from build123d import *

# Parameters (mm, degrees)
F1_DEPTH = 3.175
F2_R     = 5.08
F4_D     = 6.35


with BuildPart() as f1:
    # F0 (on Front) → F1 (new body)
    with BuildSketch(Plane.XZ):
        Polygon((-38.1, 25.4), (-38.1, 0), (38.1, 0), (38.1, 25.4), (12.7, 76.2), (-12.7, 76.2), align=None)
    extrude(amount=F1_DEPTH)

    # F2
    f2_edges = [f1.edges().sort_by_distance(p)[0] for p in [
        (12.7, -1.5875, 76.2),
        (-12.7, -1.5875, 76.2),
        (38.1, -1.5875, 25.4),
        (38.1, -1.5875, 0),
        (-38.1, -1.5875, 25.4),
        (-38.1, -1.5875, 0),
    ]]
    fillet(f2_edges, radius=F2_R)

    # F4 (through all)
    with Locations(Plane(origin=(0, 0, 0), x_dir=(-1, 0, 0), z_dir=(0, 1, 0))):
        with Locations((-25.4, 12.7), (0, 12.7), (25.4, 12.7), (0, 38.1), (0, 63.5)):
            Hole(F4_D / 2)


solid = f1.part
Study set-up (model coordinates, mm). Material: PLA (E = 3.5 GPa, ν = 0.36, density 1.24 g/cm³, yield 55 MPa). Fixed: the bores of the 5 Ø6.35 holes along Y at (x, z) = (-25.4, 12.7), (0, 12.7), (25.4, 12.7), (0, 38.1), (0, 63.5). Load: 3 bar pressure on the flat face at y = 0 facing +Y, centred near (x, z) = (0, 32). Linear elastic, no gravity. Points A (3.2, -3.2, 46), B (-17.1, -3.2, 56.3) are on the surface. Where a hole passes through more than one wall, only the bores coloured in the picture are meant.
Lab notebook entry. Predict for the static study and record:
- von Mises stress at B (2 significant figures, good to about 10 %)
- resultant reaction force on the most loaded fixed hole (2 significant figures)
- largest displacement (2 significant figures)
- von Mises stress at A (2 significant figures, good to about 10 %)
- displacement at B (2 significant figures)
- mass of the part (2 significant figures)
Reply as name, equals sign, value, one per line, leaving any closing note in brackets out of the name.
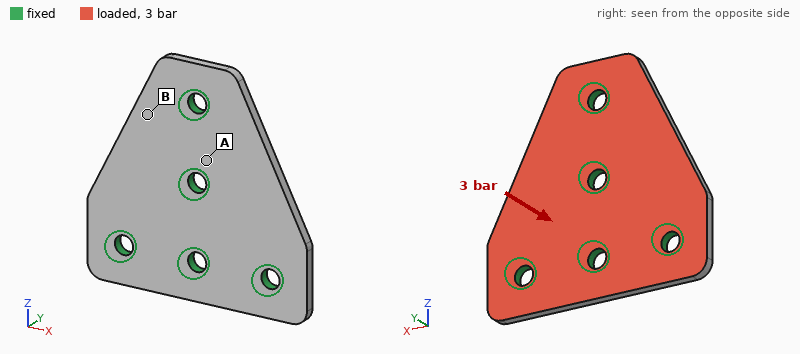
von Mises stress at B = 6.4 MPa
resultant reaction force on the most loaded fixed hole = 330 N
largest displacement = 0.86 mm
von Mises stress at A = 19 MPa
displacement at B = 0.46 mm
mass of the part = 17 g
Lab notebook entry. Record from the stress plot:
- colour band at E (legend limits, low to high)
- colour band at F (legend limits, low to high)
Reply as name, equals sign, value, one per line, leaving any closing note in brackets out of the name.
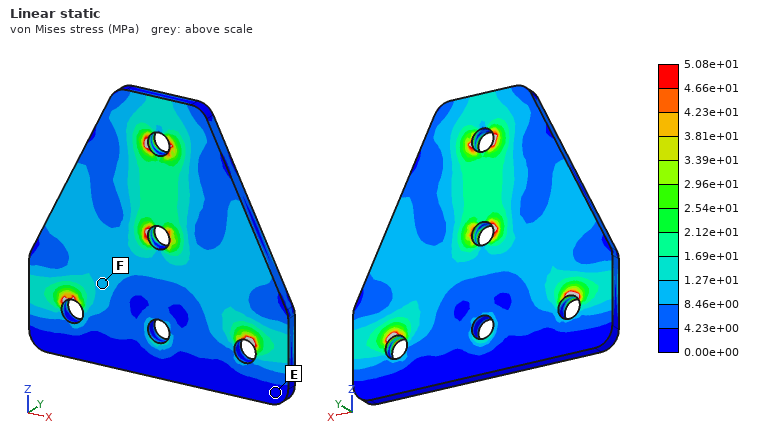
colour band at E = 0.00e+00 to 4.23e+00 MPa
colour band at F = 8.46e+00 to 1.27e+01 MPa
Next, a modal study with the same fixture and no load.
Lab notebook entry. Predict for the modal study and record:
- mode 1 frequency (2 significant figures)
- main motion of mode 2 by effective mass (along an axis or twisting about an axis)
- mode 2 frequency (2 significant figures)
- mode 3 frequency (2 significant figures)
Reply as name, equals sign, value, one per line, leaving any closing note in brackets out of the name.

mode 1 frequency = 2000 Hz
main motion of mode 2 by effective mass = along Y
mode 2 frequency = 2000 Hz
mode 3 frequency = 3600 Hz
